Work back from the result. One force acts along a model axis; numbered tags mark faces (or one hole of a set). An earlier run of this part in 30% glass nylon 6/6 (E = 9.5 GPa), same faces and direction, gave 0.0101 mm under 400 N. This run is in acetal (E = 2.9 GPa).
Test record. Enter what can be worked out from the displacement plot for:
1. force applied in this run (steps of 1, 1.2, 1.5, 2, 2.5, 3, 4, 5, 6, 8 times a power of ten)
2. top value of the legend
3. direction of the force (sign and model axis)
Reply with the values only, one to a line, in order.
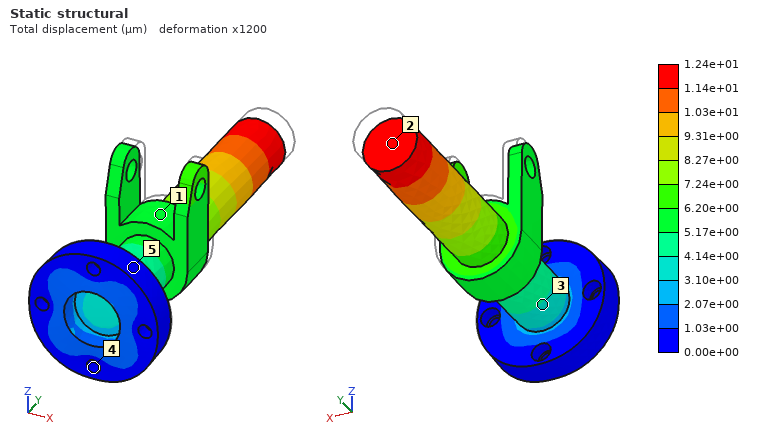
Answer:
150 N
1.24e+01 µm
-Y
